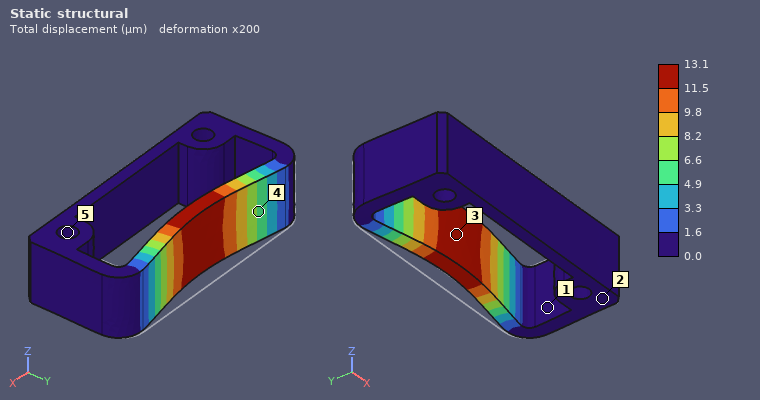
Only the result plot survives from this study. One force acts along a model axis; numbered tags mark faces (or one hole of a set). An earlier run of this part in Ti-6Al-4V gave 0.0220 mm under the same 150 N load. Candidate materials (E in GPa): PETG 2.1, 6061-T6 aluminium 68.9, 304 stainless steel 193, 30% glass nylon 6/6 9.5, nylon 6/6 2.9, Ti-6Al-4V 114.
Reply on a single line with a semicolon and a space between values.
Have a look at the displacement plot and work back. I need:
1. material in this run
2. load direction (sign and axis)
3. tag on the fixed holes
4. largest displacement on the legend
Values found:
304 stainless steel; -Y; 5; 13.1 µm
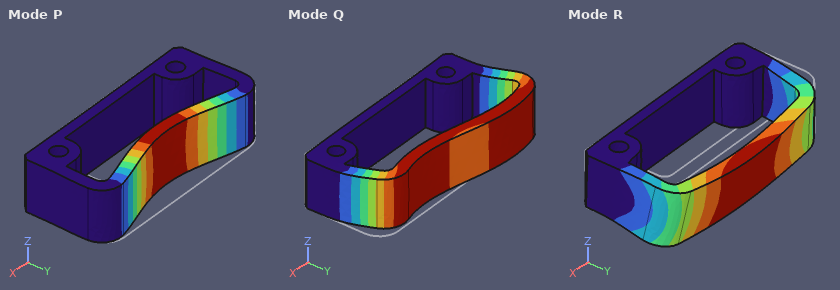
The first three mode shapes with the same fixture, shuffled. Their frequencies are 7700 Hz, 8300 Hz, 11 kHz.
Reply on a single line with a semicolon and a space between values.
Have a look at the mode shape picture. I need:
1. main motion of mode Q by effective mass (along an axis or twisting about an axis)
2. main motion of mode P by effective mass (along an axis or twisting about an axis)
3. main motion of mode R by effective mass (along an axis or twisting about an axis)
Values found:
along X; along Y; along Z
